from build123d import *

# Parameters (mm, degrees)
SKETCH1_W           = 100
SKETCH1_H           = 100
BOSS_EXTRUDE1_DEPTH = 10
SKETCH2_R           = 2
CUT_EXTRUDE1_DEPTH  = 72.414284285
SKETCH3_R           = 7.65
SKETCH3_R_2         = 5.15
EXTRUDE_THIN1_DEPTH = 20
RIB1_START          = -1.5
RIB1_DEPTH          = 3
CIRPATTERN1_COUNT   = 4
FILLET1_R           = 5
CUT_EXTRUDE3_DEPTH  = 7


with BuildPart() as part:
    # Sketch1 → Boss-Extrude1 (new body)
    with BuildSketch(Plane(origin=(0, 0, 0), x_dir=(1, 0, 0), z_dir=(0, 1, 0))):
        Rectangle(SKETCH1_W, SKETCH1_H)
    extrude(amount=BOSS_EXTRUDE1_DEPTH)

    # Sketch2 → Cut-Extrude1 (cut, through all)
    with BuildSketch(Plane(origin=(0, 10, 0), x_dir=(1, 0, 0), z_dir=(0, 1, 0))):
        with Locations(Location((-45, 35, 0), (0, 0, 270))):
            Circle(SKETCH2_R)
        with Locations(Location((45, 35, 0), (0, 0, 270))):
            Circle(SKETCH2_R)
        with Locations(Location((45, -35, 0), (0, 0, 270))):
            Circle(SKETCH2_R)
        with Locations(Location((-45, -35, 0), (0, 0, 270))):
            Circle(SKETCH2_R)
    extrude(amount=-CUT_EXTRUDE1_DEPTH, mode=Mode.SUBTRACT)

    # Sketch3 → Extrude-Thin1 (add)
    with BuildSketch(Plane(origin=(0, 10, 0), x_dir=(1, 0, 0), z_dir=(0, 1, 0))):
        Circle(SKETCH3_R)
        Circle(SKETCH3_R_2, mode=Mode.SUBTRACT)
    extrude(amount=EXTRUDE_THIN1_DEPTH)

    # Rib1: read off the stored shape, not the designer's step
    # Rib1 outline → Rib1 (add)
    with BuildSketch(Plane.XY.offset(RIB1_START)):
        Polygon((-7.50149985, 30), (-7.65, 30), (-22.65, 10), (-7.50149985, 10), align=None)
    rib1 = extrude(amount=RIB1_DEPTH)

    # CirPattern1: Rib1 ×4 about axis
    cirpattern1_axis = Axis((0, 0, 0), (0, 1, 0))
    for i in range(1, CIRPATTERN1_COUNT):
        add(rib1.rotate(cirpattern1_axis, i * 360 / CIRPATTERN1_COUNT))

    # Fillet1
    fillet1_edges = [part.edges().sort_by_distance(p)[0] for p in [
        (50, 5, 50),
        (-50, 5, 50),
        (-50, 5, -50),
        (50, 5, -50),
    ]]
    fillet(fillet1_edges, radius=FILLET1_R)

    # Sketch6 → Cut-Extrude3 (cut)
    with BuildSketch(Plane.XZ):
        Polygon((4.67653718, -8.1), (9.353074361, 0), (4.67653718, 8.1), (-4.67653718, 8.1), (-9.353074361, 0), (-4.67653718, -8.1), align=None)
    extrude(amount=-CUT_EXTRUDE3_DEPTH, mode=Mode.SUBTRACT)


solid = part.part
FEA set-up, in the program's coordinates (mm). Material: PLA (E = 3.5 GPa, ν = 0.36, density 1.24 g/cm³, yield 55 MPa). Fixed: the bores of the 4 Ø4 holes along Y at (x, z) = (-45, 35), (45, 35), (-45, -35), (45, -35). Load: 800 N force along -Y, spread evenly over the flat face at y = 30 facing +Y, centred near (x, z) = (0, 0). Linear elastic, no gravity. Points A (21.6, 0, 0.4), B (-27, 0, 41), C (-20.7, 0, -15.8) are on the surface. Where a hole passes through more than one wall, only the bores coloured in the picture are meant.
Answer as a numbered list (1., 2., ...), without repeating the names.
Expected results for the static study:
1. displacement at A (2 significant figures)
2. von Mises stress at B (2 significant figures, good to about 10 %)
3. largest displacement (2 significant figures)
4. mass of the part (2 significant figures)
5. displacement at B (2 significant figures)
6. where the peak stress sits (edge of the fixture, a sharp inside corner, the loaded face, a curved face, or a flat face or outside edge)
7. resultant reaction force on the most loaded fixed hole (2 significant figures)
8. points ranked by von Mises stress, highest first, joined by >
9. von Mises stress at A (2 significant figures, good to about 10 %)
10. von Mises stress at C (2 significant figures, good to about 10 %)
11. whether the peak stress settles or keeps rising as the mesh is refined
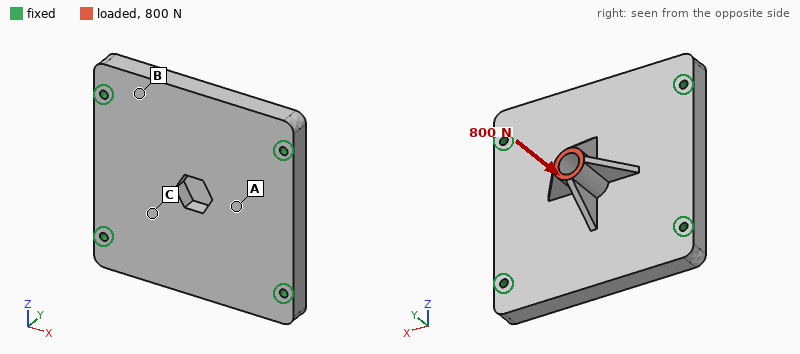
1. 0.18 mm
2. 1.3 MPa
3. 0.25 mm
4. 130 g
5. 0.058 mm
6. edge of the fixture
7. 200 N
8. A > C > B
9. 4.8 MPa
10. 2.9 MPa
11. keeps rising
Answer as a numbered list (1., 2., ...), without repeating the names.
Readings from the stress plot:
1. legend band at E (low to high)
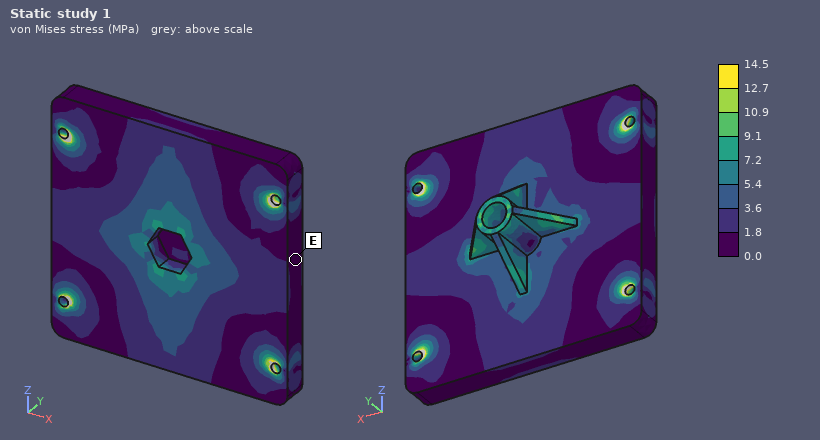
1. 0.0 to 1.8 MPa
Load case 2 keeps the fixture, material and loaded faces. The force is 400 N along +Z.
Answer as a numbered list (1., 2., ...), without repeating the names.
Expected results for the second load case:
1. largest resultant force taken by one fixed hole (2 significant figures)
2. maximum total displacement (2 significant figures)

1. 130 N
2. 0.20 mm
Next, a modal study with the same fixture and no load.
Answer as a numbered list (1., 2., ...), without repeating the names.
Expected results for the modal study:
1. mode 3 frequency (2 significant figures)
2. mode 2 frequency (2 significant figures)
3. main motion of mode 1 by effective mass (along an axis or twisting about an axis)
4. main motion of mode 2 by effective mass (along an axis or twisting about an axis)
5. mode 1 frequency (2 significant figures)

1. 2600 Hz
2. 1900 Hz
3. along Y
4. twisting about X
5. 1400 Hz
